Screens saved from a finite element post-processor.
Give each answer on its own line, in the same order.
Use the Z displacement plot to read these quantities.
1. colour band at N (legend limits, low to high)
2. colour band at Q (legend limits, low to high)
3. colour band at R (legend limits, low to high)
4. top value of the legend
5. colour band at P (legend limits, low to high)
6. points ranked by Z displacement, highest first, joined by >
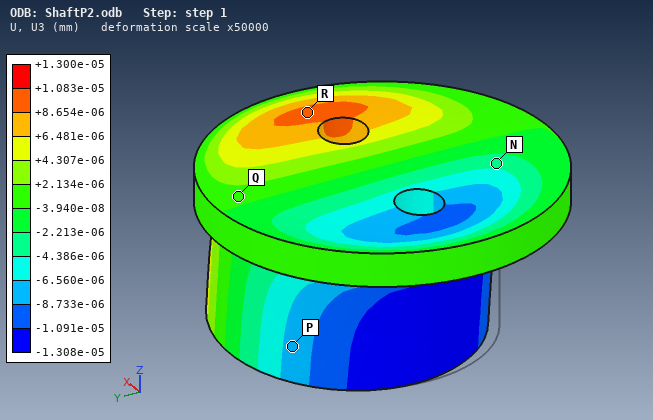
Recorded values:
-4.386e-06 to -2.213e-06 mm
-3.940e-08 to +2.134e-06 mm
+8.654e-06 to +1.083e-05 mm
+1.300e-05 mm
-8.733e-06 to -6.560e-06 mm
R > Q > N > P
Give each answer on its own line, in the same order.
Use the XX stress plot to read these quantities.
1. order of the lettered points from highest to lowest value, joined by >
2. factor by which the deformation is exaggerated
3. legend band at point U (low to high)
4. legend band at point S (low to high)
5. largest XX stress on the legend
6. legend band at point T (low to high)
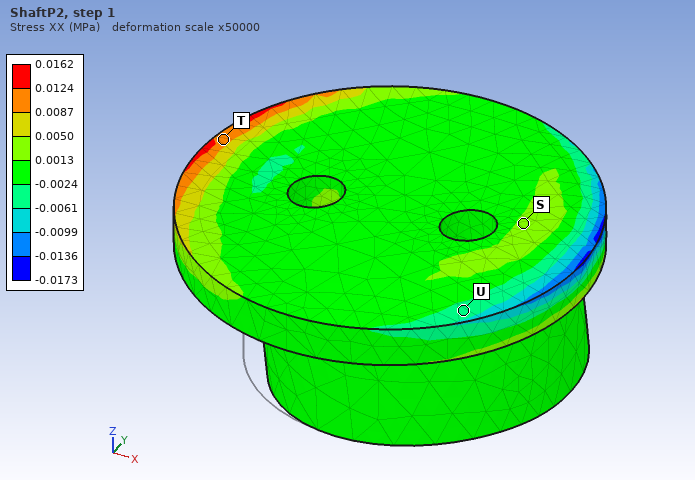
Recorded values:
T > S > U
50000
-0.0061 to -0.0024 MPa
0.0013 to 0.0050 MPa
0.0162 MPa
0.0087 to 0.0124 MPa
